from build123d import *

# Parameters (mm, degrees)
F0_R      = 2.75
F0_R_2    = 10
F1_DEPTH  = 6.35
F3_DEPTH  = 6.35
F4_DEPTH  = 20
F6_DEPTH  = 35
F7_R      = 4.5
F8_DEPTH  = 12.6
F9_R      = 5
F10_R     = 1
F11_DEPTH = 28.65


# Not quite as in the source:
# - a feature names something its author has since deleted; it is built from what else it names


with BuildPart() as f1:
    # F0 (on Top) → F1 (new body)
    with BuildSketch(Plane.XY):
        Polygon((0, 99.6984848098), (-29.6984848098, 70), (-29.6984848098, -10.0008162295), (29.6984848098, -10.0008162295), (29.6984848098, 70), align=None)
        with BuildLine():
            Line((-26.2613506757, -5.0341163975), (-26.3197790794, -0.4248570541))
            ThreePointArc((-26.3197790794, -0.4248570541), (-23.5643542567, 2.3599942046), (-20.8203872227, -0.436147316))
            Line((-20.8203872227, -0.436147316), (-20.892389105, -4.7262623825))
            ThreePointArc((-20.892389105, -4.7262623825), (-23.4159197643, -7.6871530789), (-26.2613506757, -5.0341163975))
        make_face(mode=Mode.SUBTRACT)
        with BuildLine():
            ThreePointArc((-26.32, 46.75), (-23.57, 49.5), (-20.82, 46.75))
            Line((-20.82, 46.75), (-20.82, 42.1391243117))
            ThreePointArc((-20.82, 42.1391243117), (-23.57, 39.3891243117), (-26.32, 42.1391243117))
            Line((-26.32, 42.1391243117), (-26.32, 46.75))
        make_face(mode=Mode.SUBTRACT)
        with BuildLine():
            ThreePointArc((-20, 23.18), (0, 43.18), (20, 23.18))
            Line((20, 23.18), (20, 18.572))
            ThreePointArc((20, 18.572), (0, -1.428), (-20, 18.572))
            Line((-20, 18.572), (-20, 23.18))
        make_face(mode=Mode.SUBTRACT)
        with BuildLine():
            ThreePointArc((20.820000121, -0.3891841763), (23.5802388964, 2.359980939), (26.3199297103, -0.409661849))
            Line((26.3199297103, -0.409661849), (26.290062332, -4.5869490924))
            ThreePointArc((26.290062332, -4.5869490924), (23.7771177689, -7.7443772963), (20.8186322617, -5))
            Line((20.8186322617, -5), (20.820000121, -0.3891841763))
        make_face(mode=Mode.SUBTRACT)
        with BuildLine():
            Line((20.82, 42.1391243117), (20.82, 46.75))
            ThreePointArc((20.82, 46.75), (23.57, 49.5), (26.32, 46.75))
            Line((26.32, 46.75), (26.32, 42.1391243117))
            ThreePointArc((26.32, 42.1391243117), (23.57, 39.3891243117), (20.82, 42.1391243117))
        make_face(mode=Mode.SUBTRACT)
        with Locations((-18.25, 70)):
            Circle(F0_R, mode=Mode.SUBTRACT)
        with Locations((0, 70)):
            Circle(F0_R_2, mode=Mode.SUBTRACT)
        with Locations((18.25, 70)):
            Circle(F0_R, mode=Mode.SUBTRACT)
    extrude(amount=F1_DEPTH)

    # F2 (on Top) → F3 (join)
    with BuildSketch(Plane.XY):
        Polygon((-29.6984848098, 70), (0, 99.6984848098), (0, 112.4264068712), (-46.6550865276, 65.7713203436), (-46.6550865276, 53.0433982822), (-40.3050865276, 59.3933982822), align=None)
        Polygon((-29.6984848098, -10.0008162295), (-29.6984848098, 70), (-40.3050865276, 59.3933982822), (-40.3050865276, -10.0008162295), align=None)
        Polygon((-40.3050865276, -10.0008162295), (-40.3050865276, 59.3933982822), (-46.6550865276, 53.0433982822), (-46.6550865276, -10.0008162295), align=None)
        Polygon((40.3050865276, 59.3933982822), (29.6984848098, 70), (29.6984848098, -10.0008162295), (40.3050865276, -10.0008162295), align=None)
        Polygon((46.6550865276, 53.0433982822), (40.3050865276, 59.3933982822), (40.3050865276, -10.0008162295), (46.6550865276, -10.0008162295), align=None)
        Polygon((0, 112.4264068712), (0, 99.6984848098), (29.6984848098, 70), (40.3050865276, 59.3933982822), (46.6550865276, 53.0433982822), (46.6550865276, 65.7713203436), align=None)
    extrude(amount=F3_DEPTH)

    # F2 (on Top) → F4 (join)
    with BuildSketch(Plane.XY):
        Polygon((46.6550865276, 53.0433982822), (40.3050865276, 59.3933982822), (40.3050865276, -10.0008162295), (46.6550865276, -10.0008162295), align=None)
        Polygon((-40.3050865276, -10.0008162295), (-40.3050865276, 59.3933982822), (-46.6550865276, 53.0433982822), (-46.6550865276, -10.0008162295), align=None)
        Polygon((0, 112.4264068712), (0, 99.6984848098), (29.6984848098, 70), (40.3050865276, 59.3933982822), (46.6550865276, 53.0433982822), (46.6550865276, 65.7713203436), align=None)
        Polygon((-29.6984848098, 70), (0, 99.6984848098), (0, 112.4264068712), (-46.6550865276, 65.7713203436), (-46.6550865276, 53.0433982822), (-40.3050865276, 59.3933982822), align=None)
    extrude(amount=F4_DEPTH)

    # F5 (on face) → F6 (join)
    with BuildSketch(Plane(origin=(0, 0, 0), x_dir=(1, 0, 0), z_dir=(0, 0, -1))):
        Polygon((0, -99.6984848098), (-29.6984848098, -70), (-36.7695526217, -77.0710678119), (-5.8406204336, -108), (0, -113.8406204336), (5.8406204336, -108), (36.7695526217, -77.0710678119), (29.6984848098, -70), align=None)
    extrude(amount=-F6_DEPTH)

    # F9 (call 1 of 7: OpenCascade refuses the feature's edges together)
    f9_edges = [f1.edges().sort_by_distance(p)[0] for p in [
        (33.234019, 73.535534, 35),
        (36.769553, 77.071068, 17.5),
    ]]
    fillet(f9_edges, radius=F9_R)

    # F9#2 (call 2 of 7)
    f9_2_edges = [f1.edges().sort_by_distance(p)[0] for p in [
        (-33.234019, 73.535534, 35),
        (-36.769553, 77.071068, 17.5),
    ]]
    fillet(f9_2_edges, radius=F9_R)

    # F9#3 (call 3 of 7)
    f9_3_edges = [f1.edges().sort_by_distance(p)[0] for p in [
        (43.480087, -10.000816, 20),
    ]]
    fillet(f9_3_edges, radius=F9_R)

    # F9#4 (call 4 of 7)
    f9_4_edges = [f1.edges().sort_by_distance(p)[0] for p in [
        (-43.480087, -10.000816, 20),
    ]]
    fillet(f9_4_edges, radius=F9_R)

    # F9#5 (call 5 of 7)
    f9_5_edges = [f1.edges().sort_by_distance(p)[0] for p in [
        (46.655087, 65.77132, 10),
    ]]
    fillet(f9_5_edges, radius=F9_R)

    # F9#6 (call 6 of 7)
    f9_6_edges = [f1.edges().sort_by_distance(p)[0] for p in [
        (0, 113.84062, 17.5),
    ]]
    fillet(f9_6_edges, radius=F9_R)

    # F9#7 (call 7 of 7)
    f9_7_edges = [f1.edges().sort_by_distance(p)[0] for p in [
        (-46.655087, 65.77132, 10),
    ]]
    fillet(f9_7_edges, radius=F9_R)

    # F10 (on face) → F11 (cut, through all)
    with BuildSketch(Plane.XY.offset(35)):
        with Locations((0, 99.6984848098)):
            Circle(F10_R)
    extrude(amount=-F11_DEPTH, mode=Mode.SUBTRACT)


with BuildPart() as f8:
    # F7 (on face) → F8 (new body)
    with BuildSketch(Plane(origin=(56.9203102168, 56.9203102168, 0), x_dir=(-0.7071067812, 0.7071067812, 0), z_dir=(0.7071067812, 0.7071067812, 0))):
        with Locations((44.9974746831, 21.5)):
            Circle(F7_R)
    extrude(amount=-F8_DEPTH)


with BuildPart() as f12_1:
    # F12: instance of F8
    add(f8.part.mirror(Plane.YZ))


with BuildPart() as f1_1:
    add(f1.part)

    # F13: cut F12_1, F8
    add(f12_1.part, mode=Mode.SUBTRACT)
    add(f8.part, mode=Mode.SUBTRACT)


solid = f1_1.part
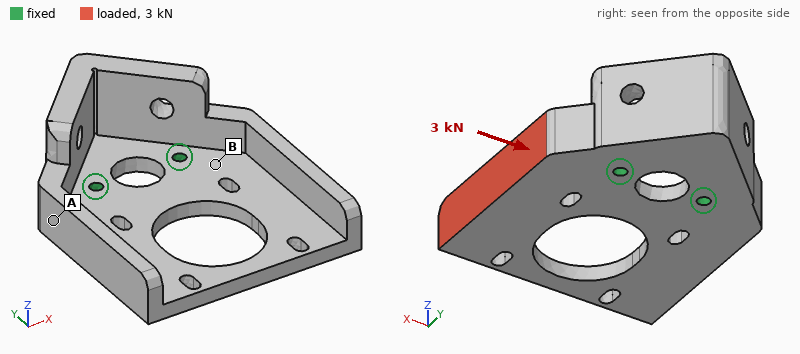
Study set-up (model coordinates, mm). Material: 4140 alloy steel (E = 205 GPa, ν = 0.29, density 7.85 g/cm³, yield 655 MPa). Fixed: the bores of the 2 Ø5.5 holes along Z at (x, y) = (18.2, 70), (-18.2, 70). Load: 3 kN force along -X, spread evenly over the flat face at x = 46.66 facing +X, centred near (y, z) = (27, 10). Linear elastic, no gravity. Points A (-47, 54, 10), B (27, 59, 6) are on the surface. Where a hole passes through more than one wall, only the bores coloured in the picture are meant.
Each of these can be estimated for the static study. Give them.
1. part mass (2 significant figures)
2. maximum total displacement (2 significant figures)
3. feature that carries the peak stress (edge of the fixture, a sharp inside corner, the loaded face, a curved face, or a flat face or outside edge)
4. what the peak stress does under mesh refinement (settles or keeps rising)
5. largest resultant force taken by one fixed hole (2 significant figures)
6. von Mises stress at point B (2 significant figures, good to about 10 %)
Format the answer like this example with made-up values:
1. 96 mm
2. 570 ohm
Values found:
1. 690 g
2. 78 µm
3. edge of the fixture
4. keeps rising
5. 3.3 kN
6. 30 MPa
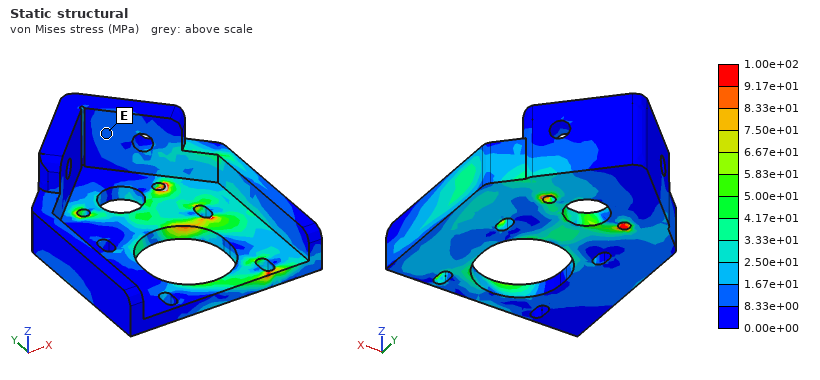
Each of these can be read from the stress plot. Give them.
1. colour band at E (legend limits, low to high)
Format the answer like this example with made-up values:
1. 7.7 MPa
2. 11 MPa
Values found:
1. 8.33e+00 to 1.67e+01 MPa
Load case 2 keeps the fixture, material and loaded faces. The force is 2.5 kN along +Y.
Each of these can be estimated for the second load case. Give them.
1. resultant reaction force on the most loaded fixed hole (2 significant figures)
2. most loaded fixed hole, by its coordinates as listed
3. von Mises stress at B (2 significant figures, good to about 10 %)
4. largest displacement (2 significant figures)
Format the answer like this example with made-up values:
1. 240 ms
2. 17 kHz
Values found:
1. 4.0 kN
2. (18.2, 70)
3. 27 MPa
4. 52 µm
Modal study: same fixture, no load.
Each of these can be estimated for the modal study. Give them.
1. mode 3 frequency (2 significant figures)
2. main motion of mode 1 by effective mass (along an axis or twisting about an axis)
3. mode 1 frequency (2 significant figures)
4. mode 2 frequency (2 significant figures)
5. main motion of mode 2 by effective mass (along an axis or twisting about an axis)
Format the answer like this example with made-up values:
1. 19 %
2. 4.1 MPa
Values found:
1. 2800 Hz
2. along Z
3. 970 Hz
4. 1800 Hz
5. twisting about Y
